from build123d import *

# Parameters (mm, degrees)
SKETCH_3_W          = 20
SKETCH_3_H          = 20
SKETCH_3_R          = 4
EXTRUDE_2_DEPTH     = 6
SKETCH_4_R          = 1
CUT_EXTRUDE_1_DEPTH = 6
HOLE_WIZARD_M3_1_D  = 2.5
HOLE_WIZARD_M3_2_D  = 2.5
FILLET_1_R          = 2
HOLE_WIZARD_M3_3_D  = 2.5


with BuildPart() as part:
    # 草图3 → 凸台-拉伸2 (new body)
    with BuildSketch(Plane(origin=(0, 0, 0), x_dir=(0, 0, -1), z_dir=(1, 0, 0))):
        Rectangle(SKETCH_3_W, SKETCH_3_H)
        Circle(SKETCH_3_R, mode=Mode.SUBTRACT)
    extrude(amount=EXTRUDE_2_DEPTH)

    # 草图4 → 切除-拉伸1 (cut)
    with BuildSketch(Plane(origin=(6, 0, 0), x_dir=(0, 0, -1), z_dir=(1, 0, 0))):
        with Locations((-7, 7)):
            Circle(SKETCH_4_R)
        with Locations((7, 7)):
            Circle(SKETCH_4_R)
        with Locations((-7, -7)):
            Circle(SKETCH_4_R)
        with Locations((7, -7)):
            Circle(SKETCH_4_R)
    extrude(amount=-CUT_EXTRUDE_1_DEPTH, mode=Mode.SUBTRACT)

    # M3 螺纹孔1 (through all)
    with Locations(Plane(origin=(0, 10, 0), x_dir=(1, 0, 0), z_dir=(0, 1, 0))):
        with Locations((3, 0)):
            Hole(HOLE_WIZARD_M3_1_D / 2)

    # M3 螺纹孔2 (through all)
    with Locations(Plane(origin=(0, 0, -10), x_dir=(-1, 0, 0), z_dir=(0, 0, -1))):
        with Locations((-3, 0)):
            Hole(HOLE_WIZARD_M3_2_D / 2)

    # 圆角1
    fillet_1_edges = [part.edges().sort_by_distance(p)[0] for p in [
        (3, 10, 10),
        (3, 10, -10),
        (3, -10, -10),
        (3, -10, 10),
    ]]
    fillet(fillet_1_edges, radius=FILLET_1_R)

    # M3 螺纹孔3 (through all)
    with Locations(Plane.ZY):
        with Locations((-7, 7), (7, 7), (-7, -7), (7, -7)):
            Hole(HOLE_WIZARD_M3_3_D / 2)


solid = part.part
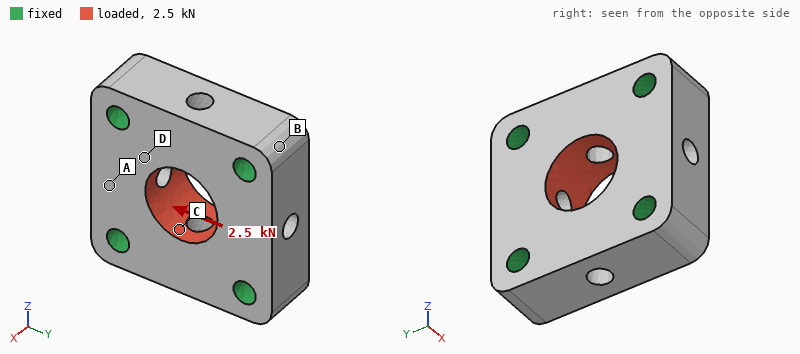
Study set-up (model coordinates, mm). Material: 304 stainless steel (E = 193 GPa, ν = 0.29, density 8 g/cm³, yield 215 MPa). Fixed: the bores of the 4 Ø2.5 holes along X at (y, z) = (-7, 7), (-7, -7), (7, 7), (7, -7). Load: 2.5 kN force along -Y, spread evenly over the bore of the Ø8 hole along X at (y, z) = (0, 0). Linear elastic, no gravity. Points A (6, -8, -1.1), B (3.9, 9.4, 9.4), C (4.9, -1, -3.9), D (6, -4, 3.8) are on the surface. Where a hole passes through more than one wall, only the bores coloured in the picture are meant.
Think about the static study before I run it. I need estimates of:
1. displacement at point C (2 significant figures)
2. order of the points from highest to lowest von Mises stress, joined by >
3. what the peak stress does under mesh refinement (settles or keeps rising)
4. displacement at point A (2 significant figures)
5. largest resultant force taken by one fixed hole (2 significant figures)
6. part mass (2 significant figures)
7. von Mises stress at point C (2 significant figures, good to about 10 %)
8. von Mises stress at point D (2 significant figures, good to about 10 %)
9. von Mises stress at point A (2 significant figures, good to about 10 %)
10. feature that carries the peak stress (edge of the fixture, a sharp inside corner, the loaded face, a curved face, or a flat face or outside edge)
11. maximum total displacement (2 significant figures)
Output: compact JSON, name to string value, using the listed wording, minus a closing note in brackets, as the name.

{"displacement at point C": "0.70 µm", "order of the points from highest to lowest von Mises stress, joined by >": "C > D > A > B", "what the peak stress does under mesh refinement": "keeps rising", "displacement at point A": "0.87 µm", "largest resultant force taken by one fixed hole": "660 N", "part mass": "15 g", "von Mises stress at point C": "37 MPa", "von Mises stress at point D": "20 MPa", "von Mises stress at point A": "11 MPa", "feature that carries the peak stress": "edge of the fixture", "maximum total displacement": "1.2 µm"}
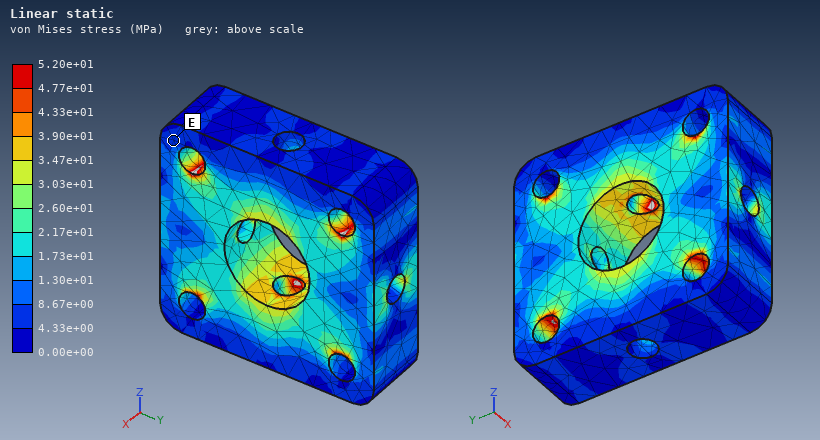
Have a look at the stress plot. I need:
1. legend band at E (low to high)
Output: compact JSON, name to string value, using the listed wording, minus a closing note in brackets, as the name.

{"legend band at E": "4.33e+00 to 8.67e+00 MPa"}
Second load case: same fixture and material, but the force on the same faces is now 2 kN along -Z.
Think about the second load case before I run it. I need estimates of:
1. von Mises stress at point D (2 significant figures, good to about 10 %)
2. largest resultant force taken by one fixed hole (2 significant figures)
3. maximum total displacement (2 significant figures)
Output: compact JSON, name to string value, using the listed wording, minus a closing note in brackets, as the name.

{"von Mises stress at point D": "16 MPa", "largest resultant force taken by one fixed hole": "530 N", "maximum total displacement": "0.94 µm"}
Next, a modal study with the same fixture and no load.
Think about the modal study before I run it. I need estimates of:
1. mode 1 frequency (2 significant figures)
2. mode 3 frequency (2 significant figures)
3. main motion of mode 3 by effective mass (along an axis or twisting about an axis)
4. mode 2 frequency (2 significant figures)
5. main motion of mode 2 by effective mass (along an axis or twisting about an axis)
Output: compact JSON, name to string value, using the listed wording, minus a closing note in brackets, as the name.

{"mode 1 frequency": "80 kHz", "mode 3 frequency": "100 kHz", "main motion of mode 3 by effective mass": "twisting about Z", "mode 2 frequency": "88 kHz", "main motion of mode 2 by effective mass": "along X"}
